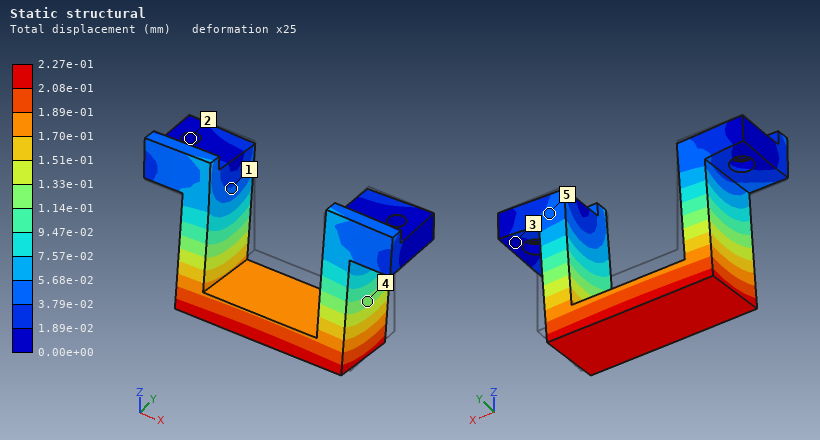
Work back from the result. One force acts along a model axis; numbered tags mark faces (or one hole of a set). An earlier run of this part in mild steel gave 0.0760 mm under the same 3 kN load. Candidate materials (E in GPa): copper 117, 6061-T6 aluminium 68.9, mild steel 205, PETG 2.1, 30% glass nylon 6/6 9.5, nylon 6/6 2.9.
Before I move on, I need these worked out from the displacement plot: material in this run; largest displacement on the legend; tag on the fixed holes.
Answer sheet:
6061-T6 aluminium
2.27e-01 mm
2
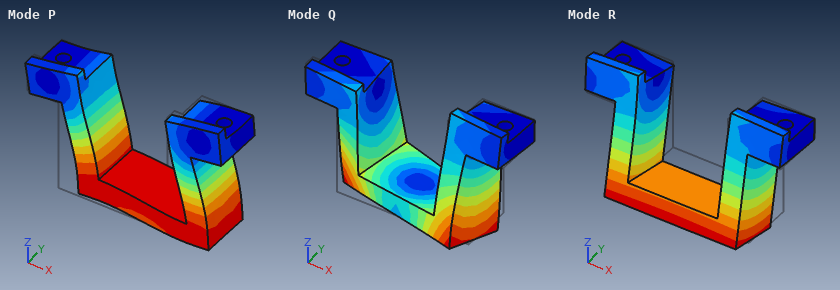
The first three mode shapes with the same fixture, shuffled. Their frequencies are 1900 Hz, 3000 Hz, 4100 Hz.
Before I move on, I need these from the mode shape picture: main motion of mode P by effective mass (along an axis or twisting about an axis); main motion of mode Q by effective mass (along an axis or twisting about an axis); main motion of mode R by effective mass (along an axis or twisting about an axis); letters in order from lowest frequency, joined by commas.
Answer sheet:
along X
twisting about Z
along Y
R, P, Q
